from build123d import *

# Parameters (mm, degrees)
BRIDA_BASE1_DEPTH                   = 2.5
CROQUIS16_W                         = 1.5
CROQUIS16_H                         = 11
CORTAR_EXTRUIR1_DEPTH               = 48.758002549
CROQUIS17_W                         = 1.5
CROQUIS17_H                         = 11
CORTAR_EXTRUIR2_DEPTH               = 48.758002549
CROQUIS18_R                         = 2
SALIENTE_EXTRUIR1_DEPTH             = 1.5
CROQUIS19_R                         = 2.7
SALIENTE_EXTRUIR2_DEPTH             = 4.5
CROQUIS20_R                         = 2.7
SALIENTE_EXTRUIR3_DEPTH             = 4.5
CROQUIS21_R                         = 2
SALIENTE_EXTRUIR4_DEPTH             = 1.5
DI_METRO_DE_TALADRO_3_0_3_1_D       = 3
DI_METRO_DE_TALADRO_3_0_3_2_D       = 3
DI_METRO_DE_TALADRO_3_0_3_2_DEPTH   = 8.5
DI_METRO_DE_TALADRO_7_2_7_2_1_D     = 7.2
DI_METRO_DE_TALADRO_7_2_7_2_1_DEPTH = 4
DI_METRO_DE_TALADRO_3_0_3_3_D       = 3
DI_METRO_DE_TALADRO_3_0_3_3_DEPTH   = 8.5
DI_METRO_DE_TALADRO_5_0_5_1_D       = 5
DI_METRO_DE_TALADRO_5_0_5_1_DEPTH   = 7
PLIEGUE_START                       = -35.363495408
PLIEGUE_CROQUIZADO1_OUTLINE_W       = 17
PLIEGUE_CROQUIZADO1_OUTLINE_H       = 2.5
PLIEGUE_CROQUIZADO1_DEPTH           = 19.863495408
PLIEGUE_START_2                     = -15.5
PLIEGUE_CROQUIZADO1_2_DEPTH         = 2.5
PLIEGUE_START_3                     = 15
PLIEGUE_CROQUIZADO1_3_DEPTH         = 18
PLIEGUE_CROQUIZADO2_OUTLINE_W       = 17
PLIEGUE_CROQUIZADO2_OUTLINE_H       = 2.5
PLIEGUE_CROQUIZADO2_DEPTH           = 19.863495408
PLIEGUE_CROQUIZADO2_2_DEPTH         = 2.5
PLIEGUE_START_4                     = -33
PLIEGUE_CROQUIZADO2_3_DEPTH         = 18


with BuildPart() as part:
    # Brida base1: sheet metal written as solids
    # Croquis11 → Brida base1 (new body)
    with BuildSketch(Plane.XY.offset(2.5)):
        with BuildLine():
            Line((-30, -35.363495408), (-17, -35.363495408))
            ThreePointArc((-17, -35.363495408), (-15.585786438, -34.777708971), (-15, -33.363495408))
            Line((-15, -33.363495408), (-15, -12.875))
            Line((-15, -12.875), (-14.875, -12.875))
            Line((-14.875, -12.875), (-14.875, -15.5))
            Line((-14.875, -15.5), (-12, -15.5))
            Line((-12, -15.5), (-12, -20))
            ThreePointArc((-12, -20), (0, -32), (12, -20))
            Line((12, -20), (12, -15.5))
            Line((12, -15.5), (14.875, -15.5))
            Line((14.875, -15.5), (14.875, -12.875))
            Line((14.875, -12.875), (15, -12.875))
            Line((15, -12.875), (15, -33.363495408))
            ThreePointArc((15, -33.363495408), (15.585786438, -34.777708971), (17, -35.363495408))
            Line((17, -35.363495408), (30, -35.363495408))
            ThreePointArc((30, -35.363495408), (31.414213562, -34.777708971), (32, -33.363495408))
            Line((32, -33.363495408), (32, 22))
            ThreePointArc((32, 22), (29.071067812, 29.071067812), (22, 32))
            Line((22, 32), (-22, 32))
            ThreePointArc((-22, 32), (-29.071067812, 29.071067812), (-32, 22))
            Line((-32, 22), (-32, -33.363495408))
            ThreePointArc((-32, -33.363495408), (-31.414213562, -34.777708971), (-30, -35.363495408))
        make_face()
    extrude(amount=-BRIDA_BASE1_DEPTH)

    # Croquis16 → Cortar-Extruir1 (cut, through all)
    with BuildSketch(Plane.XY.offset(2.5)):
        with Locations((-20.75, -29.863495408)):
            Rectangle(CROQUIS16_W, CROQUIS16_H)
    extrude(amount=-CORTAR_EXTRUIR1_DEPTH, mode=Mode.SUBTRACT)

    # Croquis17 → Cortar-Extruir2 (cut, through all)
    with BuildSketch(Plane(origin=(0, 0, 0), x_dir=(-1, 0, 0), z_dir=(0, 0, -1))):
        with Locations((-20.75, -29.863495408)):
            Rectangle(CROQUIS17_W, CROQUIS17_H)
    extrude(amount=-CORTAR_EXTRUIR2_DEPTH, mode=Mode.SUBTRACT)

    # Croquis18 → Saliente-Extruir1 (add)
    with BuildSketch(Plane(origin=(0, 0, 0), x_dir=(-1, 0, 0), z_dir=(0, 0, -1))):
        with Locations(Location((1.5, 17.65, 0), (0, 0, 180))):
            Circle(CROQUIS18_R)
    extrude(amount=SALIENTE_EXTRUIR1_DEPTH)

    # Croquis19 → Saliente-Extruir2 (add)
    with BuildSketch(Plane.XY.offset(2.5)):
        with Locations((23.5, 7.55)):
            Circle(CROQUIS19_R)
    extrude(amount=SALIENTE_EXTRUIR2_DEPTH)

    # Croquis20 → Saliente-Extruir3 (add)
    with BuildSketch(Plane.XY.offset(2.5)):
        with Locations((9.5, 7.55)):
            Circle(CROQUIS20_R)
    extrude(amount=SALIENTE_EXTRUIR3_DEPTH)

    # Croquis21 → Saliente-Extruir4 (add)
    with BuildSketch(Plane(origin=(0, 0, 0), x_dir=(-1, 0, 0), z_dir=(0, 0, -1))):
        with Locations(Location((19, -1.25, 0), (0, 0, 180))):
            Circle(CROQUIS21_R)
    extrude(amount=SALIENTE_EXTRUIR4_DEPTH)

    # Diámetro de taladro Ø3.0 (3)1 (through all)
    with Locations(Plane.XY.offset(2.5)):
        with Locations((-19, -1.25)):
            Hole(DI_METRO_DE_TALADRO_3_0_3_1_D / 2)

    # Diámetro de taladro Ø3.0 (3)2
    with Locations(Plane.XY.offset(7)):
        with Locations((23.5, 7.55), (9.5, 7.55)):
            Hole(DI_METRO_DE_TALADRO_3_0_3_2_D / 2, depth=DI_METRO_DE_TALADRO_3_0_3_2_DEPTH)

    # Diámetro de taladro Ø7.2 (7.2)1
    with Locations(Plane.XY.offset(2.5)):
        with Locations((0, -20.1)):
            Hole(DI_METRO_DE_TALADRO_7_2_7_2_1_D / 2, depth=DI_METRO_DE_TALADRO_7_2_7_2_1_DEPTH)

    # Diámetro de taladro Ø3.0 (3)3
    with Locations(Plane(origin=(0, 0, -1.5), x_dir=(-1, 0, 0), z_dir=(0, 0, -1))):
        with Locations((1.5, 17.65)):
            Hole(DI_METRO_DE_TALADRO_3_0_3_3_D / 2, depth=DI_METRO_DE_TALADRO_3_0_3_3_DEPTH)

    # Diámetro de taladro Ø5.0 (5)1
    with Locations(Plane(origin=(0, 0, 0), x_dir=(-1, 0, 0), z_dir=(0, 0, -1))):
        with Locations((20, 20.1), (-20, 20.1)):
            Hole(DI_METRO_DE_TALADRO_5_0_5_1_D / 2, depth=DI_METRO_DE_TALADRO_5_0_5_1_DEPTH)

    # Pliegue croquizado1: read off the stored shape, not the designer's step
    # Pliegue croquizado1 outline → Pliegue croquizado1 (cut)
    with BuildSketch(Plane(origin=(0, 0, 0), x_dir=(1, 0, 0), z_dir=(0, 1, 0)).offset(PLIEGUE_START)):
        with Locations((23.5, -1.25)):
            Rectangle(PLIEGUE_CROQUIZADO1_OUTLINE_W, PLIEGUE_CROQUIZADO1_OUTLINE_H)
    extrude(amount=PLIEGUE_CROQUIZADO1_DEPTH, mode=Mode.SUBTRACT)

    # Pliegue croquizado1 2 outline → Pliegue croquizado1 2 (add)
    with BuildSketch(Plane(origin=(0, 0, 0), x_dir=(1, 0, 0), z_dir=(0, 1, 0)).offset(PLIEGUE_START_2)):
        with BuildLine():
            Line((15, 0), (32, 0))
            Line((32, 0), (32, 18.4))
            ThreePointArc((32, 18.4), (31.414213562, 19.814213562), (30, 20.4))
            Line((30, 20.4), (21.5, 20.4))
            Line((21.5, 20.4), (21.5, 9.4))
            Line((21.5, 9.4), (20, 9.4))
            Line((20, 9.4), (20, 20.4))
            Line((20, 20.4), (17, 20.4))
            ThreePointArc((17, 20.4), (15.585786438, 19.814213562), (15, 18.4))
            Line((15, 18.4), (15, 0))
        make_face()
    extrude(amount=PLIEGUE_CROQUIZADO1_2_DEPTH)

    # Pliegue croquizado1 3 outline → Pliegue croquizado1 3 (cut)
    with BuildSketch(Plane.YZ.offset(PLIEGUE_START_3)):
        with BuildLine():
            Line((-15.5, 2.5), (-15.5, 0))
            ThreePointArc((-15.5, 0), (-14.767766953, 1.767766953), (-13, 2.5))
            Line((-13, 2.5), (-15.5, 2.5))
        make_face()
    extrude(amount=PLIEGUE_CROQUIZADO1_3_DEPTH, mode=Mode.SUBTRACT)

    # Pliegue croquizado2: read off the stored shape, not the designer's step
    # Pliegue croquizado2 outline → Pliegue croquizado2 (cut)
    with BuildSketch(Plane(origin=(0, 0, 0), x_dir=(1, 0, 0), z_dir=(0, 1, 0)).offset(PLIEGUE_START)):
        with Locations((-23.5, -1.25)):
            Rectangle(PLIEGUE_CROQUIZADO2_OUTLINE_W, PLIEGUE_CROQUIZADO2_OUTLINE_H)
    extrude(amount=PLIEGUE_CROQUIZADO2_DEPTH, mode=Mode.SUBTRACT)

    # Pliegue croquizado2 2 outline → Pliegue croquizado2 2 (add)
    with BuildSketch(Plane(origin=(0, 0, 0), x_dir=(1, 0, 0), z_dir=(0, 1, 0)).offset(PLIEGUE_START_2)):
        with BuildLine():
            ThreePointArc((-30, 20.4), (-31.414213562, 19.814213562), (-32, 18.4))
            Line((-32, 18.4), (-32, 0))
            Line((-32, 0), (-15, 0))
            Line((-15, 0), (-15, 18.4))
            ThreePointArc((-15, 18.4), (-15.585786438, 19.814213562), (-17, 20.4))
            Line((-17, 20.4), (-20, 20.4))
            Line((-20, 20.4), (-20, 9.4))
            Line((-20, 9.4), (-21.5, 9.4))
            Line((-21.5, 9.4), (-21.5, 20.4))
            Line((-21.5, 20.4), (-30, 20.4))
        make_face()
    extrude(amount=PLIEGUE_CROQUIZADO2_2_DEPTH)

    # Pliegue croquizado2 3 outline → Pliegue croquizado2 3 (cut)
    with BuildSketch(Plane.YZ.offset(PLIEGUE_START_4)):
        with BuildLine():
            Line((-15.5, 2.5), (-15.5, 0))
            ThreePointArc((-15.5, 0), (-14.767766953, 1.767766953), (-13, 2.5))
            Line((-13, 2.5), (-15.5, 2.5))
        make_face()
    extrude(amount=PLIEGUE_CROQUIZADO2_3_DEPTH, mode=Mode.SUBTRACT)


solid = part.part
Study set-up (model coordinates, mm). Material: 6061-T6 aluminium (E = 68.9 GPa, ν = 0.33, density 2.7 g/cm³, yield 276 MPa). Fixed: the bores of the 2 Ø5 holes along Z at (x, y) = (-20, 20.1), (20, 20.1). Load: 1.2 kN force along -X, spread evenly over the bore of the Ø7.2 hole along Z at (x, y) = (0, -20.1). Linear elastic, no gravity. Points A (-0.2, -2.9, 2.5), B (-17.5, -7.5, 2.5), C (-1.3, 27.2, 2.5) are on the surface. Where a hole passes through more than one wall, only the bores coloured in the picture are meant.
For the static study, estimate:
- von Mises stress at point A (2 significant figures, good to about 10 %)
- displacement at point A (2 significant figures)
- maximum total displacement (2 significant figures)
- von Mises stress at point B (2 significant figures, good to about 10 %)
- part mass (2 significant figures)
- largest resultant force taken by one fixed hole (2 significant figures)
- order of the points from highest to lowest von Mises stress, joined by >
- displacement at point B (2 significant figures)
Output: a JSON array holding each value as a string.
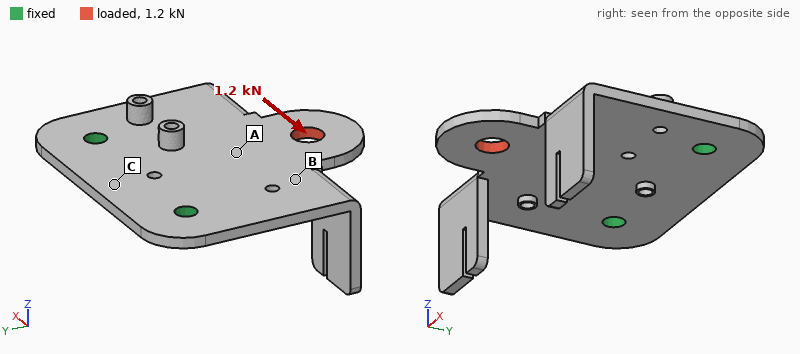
["15 MPa", "13 µm", "42 µm", "21 MPa", "26 g", "1.3 kN", "B > A > C", "18 µm"]
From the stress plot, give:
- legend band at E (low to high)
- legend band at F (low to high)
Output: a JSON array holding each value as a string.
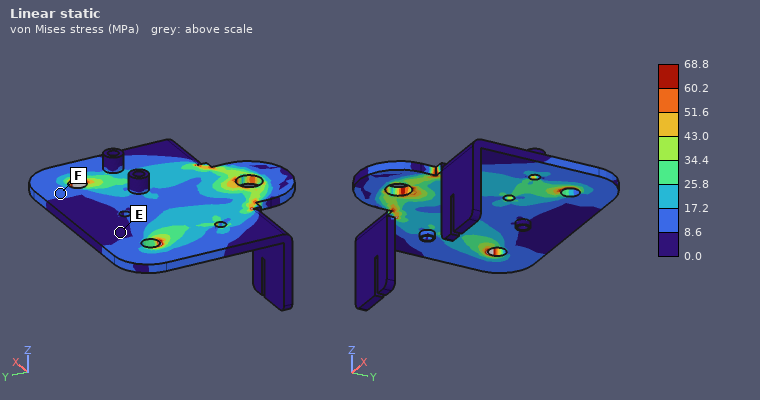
["0.0 to 8.6 MPa", "8.6 to 17.2 MPa"]
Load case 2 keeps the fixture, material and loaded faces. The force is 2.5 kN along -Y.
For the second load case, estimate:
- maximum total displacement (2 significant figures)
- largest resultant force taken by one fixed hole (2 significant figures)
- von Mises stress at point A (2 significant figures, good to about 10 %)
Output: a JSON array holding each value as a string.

["27 µm", "1.3 kN", "29 MPa"]
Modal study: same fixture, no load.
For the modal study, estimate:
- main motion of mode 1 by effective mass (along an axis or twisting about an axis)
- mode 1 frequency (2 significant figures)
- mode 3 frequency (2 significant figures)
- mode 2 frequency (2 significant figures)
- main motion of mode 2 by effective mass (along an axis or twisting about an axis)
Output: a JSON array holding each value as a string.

["along Z", "880 Hz", "2200 Hz", "1500 Hz", "twisting about Y"]
